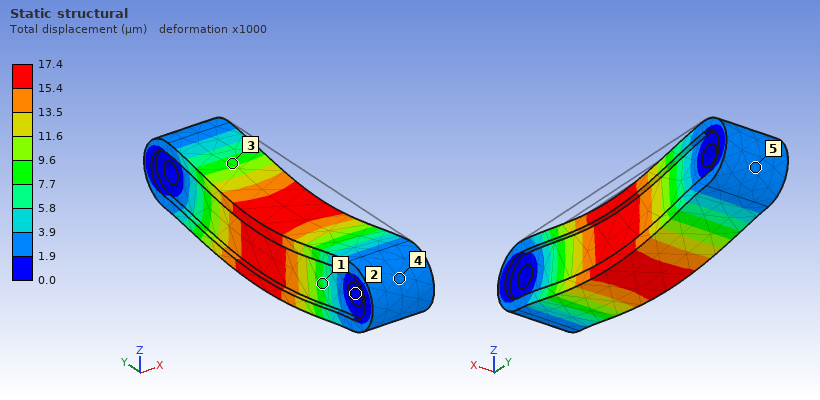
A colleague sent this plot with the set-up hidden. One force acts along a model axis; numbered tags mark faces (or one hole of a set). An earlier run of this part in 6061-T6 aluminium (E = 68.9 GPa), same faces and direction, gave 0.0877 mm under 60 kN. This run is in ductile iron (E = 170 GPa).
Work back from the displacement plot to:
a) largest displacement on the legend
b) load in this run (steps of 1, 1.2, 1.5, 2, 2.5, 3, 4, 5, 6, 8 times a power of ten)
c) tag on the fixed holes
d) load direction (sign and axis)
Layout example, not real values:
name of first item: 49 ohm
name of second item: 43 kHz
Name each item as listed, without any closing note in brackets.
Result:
largest displacement on the legend: 17.4 µm
load in this run: 30 kN
tag on the fixed holes: 2
load direction: -Z
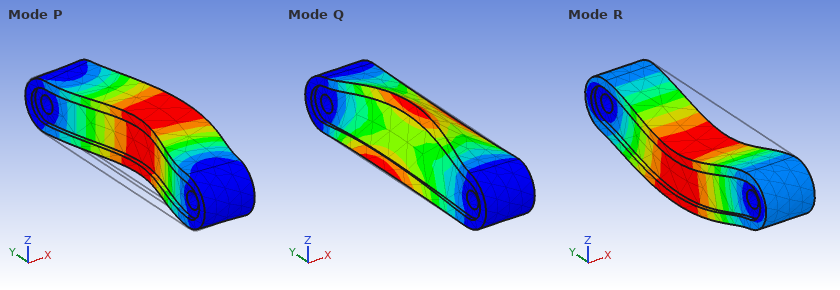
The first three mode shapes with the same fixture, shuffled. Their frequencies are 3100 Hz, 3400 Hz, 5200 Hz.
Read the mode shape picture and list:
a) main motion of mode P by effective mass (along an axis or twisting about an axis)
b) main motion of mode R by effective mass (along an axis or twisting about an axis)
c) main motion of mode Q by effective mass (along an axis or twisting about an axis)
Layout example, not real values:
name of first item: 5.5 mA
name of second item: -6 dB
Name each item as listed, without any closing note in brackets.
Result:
main motion of mode P by effective mass: along X
main motion of mode R by effective mass: along Z
main motion of mode Q by effective mass: twisting about Y
